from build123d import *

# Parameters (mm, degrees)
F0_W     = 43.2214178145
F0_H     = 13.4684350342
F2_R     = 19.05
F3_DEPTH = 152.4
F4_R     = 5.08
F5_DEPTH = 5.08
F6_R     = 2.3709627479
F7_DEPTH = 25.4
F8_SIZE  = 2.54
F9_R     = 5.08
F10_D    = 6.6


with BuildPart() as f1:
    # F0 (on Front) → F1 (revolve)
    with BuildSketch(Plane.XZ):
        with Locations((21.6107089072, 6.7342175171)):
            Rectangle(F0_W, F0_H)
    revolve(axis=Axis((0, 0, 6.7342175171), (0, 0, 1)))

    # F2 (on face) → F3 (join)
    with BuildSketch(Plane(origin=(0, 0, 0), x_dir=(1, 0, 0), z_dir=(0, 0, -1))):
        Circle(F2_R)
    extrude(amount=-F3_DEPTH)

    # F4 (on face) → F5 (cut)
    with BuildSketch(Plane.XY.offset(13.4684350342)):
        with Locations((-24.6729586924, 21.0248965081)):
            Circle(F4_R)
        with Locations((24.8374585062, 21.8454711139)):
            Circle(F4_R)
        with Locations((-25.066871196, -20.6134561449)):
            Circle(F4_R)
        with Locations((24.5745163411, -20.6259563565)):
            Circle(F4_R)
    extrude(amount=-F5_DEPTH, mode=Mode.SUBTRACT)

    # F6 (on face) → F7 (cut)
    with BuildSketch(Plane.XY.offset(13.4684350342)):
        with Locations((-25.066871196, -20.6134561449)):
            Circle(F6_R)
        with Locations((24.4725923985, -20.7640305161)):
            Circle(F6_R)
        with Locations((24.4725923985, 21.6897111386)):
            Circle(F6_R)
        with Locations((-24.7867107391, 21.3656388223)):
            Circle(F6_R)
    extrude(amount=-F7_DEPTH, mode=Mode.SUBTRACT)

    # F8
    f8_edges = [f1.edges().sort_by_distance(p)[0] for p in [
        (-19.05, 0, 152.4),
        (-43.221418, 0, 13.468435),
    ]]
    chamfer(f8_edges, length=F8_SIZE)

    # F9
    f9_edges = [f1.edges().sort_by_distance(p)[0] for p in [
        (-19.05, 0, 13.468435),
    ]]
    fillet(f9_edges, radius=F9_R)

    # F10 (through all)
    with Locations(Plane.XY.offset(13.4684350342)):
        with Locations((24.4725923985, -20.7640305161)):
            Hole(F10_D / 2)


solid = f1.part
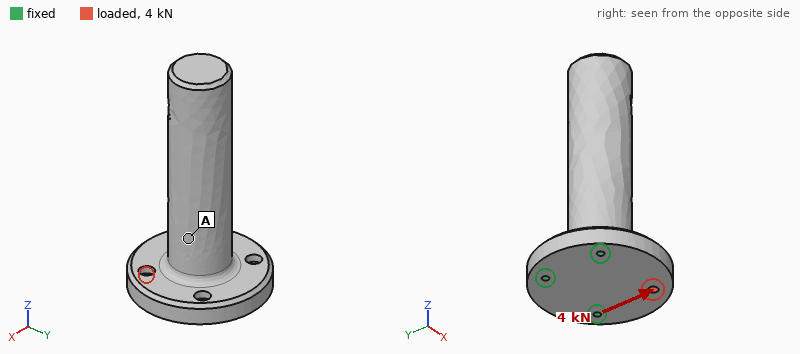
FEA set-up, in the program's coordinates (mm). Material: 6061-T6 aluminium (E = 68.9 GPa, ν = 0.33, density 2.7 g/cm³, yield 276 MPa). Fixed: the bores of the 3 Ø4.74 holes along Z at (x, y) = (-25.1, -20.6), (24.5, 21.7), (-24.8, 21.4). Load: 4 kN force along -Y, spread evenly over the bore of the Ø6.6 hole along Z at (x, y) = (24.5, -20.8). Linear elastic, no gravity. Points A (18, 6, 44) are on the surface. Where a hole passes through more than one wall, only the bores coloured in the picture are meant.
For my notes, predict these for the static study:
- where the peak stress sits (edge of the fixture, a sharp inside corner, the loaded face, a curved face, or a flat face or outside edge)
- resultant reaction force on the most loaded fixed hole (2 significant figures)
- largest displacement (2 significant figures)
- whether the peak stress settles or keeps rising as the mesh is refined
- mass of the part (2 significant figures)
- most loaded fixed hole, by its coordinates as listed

edge of the fixture
3.2 kN
14 µm
keeps rising
630 g
(24.5, 21.7)
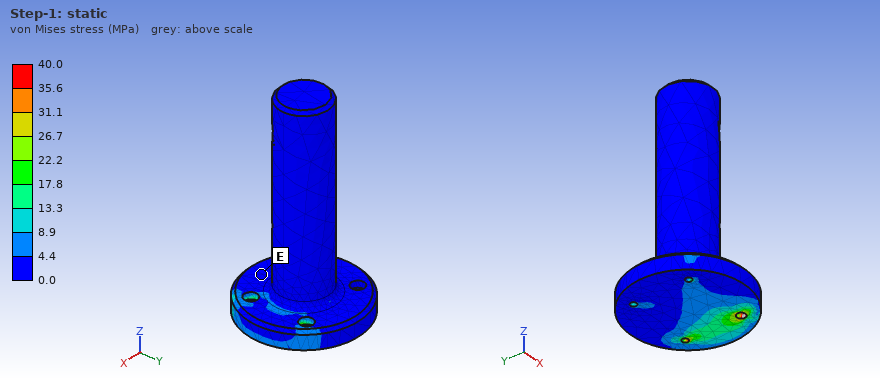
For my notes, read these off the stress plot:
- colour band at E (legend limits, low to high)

0.0 to 4.4 MPa
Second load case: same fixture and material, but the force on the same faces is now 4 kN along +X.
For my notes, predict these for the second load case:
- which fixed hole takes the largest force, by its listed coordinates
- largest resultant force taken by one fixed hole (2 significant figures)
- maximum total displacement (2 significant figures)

(-25.1, -20.6)
2.8 kN
15 µm
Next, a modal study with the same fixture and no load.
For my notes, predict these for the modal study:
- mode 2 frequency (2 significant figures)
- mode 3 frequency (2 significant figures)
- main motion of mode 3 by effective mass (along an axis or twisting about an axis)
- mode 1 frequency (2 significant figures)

1100 Hz
4200 Hz
along Z
820 Hz
